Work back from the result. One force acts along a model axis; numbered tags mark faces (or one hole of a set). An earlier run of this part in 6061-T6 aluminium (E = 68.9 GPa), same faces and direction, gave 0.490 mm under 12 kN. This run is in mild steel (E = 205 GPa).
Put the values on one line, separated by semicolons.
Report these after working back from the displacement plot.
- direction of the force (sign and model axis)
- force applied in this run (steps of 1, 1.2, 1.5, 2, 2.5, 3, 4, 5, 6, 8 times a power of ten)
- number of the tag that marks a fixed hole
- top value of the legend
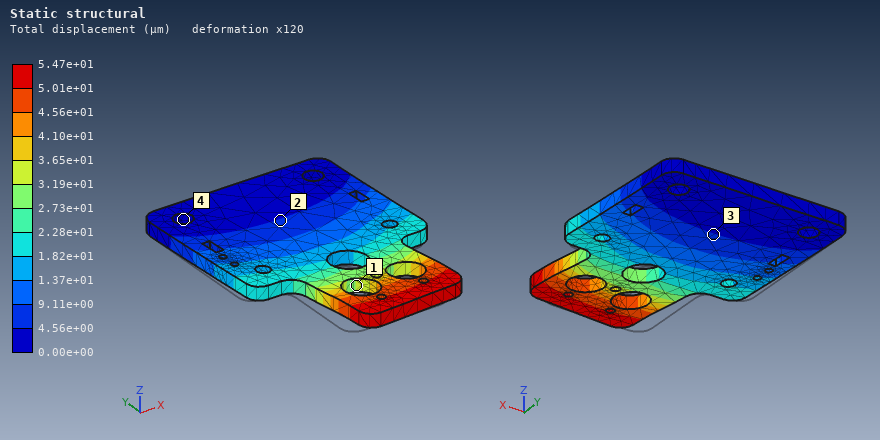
+X; 4 kN; 4; 5.47e+01 µm
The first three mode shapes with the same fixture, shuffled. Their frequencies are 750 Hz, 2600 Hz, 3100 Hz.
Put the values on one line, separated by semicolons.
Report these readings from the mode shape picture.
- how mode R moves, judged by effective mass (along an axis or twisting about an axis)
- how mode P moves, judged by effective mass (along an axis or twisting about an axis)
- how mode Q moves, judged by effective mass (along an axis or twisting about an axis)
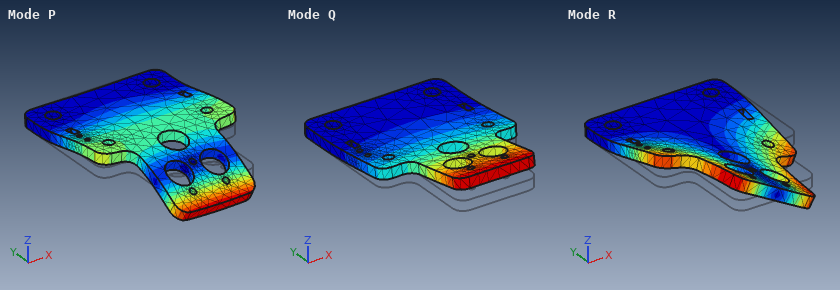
twisting about Y; along Z; along Z
